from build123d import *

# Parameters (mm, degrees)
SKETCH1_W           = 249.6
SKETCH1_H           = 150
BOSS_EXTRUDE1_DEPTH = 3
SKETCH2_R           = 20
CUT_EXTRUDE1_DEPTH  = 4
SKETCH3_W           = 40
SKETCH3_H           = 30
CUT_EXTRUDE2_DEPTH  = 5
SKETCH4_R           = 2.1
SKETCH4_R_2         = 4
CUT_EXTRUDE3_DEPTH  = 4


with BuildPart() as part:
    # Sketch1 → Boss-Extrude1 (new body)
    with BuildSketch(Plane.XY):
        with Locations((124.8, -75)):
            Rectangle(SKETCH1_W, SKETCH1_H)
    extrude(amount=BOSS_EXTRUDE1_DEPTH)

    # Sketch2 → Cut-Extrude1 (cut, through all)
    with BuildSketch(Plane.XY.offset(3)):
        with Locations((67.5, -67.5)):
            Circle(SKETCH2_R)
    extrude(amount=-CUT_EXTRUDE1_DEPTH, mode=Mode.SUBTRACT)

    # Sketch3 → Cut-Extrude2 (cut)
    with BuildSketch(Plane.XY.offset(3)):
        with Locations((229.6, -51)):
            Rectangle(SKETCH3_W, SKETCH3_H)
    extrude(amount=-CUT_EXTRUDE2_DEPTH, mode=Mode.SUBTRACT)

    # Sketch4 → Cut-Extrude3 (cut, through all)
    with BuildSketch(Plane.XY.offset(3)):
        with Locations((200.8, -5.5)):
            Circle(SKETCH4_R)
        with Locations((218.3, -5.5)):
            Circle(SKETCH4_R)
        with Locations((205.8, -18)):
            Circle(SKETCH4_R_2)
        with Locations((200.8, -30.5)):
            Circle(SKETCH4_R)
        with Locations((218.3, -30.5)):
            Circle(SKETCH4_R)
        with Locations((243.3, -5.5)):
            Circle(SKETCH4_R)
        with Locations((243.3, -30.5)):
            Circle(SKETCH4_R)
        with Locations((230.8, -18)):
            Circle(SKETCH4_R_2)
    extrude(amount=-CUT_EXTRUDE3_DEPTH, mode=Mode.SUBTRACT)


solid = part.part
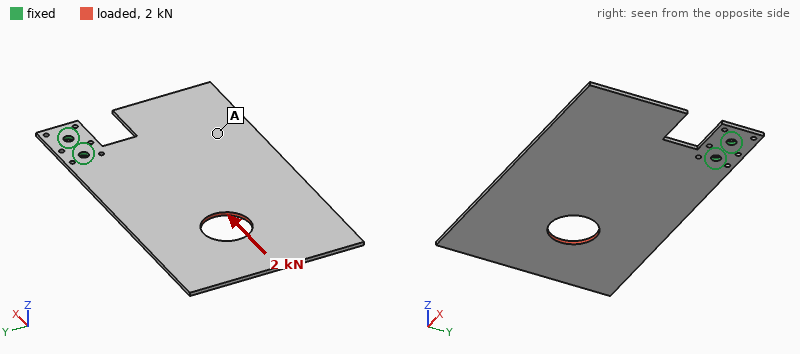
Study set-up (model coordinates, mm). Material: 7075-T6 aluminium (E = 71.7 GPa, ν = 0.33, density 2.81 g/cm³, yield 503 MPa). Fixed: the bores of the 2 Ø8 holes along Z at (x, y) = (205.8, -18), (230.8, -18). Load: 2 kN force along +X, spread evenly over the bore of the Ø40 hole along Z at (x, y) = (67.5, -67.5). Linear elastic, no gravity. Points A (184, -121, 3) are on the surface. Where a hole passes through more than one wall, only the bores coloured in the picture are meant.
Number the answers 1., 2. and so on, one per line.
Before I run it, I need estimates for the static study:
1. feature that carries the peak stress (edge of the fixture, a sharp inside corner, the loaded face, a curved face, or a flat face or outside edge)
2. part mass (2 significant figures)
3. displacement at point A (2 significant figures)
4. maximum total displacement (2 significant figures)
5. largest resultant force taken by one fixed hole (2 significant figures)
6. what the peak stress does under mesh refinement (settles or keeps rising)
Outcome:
1. a sharp inside corner
2. 290 g
3. 0.41 mm
4. 0.93 mm
5. 2.8 kN
6. keeps rising
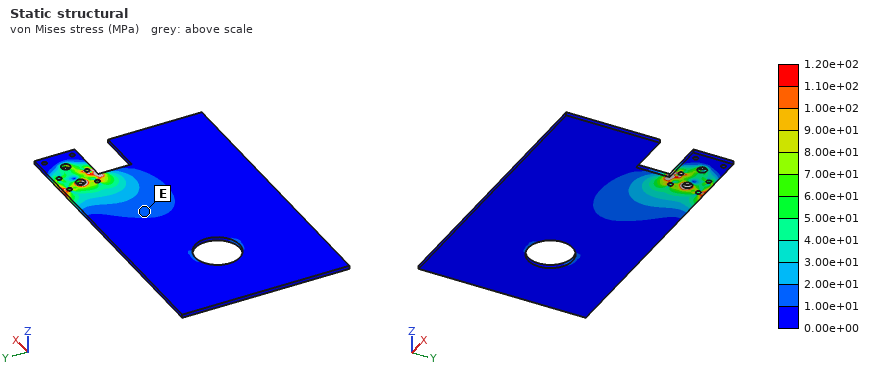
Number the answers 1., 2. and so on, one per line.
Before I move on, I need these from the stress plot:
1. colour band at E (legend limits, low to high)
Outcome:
1. 1.00e+01 to 2.00e+01 MPa
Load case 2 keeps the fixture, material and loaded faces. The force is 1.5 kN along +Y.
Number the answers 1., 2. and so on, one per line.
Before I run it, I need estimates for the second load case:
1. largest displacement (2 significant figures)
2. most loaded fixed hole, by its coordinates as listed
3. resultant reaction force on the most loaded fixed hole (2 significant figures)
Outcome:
1. 2.0 mm
2. (205.8, -18)
3. 6.8 kN
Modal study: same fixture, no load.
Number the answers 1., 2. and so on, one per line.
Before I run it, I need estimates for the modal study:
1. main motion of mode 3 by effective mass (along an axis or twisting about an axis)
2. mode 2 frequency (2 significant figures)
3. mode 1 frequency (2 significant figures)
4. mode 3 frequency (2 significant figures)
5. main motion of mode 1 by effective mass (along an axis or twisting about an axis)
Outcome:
1. along Z
2. 84 Hz
3. 38 Hz
4. 210 Hz
5. along Z
